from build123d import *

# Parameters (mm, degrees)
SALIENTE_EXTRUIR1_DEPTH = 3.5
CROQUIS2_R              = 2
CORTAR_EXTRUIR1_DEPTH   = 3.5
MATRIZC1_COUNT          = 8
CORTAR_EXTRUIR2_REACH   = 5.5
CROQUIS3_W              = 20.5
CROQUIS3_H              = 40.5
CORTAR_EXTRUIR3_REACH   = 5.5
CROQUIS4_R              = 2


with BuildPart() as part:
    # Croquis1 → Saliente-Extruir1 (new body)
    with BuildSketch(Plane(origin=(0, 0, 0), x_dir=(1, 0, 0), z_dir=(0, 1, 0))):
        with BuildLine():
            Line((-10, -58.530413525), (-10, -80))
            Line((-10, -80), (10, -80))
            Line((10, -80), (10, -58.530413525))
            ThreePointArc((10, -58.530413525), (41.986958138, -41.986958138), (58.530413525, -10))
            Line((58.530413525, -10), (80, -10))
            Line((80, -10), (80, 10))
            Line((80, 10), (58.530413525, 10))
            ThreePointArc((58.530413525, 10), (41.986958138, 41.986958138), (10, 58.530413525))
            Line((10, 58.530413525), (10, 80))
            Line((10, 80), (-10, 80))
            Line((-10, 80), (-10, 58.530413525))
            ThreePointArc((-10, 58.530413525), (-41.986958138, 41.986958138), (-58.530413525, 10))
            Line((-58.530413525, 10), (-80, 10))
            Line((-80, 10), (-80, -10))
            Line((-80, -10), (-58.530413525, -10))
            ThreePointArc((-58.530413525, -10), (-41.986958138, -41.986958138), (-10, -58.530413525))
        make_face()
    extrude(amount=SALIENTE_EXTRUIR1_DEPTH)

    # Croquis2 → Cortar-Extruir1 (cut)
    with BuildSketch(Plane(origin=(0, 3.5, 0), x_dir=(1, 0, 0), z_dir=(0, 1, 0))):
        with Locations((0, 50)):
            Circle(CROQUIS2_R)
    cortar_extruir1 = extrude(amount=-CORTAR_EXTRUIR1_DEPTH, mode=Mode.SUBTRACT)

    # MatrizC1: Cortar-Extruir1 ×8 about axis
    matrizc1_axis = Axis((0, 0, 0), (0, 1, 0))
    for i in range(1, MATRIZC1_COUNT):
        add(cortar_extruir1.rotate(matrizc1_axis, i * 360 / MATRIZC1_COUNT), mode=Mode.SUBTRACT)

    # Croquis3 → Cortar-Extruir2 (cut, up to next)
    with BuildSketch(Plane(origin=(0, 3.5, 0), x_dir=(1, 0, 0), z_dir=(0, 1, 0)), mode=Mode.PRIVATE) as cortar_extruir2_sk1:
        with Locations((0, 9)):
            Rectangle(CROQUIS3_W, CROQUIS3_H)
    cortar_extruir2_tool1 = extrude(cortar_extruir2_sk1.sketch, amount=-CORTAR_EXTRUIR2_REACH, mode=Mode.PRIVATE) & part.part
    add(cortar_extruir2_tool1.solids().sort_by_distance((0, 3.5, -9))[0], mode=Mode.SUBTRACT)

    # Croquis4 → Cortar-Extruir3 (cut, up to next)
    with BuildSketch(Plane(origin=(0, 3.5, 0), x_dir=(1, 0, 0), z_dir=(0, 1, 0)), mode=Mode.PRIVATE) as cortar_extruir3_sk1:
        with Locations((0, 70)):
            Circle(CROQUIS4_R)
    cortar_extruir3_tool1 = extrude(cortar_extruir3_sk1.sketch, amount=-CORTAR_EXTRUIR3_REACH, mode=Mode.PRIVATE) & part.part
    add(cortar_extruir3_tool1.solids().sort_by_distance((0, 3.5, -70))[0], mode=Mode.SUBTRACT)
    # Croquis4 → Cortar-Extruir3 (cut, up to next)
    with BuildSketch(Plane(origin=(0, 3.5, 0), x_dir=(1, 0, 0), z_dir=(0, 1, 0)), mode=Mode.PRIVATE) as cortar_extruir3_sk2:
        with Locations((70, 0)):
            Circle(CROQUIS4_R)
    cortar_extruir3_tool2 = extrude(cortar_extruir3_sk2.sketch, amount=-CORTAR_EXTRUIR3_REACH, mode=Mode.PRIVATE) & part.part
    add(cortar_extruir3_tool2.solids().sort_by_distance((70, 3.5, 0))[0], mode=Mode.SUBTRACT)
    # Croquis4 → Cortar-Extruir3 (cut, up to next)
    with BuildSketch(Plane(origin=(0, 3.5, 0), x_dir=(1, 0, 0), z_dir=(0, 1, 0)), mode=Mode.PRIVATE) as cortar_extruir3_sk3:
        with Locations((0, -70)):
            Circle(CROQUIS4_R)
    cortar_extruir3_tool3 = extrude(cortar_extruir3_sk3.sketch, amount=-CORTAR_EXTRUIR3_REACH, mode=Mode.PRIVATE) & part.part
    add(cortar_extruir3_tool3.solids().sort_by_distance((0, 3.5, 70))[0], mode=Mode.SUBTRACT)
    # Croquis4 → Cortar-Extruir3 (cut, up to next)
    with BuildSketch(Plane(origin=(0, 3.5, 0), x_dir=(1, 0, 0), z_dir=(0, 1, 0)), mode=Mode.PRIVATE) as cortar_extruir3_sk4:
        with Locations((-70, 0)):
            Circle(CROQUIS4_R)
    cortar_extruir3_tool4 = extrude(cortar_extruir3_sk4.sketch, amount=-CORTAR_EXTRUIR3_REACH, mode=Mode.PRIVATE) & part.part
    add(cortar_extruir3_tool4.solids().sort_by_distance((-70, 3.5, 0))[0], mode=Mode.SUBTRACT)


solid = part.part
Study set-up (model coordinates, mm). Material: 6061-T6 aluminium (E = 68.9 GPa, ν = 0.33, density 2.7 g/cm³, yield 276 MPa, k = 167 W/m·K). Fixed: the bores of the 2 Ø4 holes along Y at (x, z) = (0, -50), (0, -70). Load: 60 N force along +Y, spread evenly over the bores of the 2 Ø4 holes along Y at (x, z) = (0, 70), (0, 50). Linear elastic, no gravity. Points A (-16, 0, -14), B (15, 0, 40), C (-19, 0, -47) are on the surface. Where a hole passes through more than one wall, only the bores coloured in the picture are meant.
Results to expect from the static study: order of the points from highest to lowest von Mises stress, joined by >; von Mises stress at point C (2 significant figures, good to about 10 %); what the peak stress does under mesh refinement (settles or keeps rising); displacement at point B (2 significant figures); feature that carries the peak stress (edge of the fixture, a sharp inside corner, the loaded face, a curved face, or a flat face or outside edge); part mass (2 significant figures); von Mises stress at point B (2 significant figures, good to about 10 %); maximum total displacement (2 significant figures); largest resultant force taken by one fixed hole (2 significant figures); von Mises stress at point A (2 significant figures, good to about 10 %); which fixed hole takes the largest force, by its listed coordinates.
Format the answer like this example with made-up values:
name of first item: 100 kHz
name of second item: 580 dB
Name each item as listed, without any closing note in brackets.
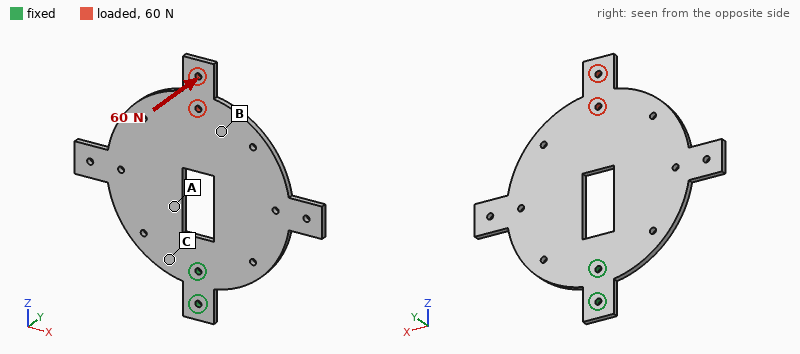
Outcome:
order of the points from highest to lowest von Mises stress, joined by >: C > A > B
von Mises stress at point C: 43 MPa
what the peak stress does under mesh refinement: keeps rising
displacement at point B: 1.4 mm
feature that carries the peak stress: edge of the fixture
part mass: 110 g
von Mises stress at point B: 9.7 MPa
maximum total displacement: 2.3 mm
largest resultant force taken by one fixed hole: 210 N
von Mises stress at point A: 29 MPa
which fixed hole takes the largest force, by its listed coordinates: (0, -50)
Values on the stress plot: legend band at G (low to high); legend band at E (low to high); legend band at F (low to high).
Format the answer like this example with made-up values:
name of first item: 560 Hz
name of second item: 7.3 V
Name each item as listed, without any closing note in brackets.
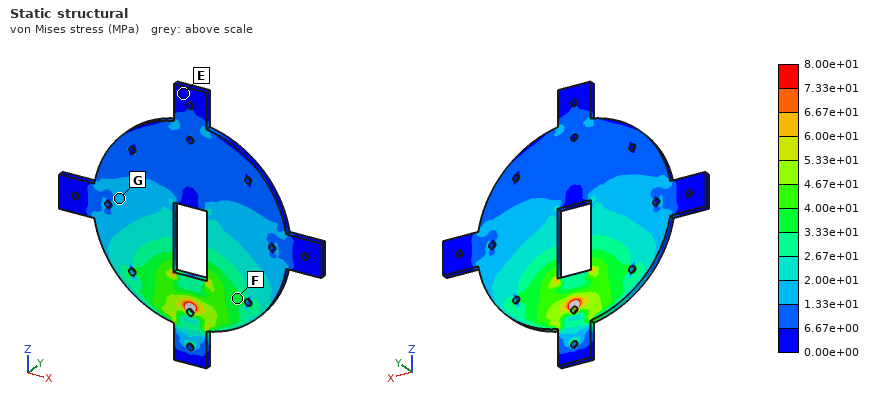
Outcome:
legend band at G: 1.33e+01 to 2.00e+01 MPa
legend band at E: 0.00e+00 to 6.67e+00 MPa
legend band at F: 3.33e+01 to 4.00e+01 MPa
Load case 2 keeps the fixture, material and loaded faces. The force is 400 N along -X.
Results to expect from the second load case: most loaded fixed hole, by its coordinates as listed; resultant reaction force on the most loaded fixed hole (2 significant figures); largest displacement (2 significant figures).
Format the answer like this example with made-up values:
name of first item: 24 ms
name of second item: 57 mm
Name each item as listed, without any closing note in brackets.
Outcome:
most loaded fixed hole, by its coordinates as listed: (0, -50)
resultant reaction force on the most loaded fixed hole: 2.2 kN
largest displacement: 0.35 mm
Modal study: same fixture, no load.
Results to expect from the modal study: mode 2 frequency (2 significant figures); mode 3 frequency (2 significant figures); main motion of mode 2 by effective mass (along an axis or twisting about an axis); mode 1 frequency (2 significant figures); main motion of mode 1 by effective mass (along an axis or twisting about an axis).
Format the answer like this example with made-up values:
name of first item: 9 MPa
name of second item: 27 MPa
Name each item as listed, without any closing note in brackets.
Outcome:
mode 2 frequency: 290 Hz
mode 3 frequency: 680 Hz
main motion of mode 2 by effective mass: twisting about Z
mode 1 frequency: 180 Hz
main motion of mode 1 by effective mass: along Y
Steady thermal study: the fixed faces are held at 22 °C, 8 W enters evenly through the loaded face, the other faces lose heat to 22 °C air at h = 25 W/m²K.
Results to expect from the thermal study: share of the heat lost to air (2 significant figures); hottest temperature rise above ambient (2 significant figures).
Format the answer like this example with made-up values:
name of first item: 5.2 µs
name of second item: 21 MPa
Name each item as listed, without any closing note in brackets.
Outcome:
share of the heat lost to air: 57 %
hottest temperature rise above ambient: 22 K
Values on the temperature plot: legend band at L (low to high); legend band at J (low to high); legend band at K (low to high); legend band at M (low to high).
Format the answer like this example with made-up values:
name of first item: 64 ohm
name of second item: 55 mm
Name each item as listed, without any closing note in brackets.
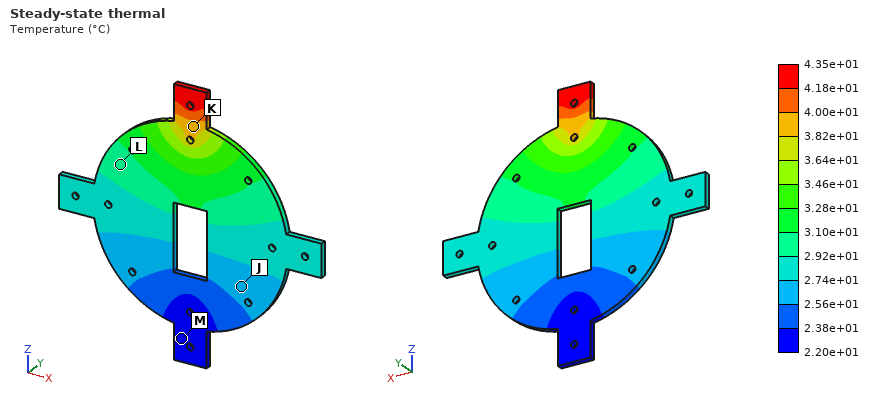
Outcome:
legend band at L: 2.92e+01 to 3.10e+01 °C
legend band at J: 2.56e+01 to 2.74e+01 °C
legend band at K: 3.82e+01 to 4.00e+01 °C
legend band at M: 2.20e+01 to 2.38e+01 °C
